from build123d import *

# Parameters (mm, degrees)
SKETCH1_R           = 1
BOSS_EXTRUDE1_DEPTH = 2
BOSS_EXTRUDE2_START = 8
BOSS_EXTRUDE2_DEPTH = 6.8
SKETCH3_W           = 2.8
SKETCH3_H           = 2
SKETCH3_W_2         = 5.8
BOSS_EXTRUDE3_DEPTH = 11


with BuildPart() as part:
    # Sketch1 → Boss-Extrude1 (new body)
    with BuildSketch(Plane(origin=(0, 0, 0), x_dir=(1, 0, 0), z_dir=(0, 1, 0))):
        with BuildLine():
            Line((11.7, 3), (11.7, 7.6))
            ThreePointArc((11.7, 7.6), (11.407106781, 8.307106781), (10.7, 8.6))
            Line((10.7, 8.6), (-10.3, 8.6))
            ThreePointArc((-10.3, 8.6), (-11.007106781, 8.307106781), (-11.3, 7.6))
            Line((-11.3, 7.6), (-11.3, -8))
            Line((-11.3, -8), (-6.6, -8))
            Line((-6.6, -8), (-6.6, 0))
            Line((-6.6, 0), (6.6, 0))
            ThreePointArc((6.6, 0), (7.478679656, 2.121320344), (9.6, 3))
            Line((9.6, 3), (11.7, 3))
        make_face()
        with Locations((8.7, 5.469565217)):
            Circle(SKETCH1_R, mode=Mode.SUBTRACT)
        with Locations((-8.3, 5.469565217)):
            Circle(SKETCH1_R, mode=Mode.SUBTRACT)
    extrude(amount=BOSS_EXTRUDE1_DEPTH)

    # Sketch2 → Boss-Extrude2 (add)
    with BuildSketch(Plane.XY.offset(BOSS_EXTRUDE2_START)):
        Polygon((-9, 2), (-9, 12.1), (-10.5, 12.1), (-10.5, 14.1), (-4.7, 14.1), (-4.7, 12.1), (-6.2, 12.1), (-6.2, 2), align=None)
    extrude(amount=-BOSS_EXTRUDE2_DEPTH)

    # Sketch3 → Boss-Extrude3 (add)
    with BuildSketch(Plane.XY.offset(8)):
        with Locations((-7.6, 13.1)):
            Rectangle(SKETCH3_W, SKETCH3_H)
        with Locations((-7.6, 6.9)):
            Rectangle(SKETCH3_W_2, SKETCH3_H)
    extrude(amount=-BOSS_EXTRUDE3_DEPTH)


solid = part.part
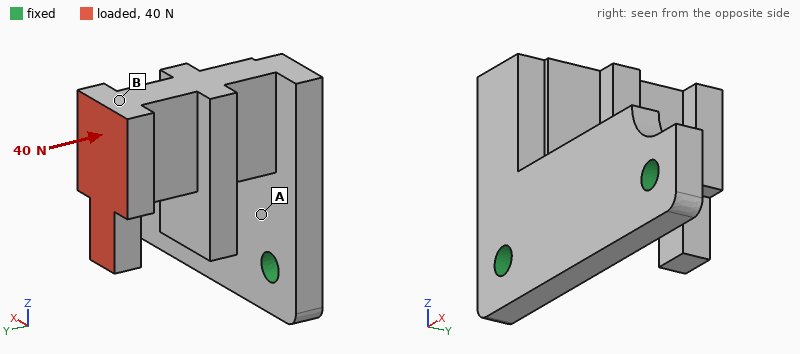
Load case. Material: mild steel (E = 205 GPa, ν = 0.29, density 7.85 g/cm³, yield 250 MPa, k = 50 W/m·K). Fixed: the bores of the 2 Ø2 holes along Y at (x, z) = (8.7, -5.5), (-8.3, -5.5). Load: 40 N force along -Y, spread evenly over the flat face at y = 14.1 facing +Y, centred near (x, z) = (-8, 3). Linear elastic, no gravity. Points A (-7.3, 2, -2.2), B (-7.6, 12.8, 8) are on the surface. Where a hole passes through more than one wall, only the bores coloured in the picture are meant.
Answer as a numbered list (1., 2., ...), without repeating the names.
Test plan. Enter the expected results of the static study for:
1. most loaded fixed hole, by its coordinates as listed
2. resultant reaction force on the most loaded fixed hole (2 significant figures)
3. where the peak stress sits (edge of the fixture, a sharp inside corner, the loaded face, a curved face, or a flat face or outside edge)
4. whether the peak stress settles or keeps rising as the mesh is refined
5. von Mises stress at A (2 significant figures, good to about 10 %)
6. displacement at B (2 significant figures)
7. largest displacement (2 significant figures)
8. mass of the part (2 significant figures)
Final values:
1. (-8.3, -5.5)
2. 41 N
3. edge of the fixture
4. keeps rising
5. 45 MPa
6. 25 µm
7. 27 µm
8. 6.4 g
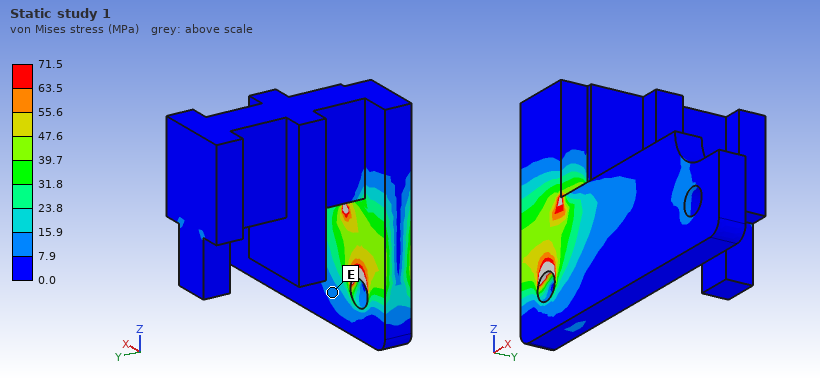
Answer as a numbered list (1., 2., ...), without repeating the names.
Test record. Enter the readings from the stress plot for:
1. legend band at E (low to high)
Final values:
1. 7.9 to 15.9 MPa
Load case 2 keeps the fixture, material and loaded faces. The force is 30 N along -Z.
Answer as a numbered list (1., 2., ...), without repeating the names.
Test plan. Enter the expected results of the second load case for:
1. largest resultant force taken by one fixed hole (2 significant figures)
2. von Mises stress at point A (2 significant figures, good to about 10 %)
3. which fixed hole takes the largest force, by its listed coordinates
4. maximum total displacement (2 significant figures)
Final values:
1. 29 N
2. 85 MPa
3. (-8.3, -5.5)
4. 62 µm
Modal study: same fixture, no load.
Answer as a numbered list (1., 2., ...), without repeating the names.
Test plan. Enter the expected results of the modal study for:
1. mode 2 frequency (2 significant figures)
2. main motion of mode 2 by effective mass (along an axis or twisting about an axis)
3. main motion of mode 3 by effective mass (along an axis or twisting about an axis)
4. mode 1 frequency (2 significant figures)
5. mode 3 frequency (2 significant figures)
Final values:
1. 3600 Hz
2. along X
3. along Y
4. 2900 Hz
5. 12 kHz
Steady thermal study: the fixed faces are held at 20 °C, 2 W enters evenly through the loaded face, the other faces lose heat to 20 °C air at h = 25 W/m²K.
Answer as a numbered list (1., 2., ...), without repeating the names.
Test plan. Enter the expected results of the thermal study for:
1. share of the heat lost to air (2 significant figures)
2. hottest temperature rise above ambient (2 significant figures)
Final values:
1. 22 %
2. 48 K
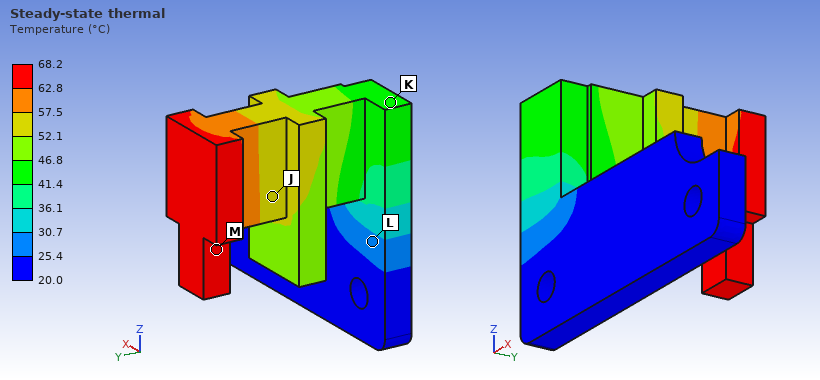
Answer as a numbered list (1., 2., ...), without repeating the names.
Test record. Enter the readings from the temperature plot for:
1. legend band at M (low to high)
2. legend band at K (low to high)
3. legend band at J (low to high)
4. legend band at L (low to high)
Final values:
1. 62.8 to 68.2 °C
2. 41.4 to 46.8 °C
3. 52.1 to 57.5 °C
4. 25.4 to 30.7 °C
